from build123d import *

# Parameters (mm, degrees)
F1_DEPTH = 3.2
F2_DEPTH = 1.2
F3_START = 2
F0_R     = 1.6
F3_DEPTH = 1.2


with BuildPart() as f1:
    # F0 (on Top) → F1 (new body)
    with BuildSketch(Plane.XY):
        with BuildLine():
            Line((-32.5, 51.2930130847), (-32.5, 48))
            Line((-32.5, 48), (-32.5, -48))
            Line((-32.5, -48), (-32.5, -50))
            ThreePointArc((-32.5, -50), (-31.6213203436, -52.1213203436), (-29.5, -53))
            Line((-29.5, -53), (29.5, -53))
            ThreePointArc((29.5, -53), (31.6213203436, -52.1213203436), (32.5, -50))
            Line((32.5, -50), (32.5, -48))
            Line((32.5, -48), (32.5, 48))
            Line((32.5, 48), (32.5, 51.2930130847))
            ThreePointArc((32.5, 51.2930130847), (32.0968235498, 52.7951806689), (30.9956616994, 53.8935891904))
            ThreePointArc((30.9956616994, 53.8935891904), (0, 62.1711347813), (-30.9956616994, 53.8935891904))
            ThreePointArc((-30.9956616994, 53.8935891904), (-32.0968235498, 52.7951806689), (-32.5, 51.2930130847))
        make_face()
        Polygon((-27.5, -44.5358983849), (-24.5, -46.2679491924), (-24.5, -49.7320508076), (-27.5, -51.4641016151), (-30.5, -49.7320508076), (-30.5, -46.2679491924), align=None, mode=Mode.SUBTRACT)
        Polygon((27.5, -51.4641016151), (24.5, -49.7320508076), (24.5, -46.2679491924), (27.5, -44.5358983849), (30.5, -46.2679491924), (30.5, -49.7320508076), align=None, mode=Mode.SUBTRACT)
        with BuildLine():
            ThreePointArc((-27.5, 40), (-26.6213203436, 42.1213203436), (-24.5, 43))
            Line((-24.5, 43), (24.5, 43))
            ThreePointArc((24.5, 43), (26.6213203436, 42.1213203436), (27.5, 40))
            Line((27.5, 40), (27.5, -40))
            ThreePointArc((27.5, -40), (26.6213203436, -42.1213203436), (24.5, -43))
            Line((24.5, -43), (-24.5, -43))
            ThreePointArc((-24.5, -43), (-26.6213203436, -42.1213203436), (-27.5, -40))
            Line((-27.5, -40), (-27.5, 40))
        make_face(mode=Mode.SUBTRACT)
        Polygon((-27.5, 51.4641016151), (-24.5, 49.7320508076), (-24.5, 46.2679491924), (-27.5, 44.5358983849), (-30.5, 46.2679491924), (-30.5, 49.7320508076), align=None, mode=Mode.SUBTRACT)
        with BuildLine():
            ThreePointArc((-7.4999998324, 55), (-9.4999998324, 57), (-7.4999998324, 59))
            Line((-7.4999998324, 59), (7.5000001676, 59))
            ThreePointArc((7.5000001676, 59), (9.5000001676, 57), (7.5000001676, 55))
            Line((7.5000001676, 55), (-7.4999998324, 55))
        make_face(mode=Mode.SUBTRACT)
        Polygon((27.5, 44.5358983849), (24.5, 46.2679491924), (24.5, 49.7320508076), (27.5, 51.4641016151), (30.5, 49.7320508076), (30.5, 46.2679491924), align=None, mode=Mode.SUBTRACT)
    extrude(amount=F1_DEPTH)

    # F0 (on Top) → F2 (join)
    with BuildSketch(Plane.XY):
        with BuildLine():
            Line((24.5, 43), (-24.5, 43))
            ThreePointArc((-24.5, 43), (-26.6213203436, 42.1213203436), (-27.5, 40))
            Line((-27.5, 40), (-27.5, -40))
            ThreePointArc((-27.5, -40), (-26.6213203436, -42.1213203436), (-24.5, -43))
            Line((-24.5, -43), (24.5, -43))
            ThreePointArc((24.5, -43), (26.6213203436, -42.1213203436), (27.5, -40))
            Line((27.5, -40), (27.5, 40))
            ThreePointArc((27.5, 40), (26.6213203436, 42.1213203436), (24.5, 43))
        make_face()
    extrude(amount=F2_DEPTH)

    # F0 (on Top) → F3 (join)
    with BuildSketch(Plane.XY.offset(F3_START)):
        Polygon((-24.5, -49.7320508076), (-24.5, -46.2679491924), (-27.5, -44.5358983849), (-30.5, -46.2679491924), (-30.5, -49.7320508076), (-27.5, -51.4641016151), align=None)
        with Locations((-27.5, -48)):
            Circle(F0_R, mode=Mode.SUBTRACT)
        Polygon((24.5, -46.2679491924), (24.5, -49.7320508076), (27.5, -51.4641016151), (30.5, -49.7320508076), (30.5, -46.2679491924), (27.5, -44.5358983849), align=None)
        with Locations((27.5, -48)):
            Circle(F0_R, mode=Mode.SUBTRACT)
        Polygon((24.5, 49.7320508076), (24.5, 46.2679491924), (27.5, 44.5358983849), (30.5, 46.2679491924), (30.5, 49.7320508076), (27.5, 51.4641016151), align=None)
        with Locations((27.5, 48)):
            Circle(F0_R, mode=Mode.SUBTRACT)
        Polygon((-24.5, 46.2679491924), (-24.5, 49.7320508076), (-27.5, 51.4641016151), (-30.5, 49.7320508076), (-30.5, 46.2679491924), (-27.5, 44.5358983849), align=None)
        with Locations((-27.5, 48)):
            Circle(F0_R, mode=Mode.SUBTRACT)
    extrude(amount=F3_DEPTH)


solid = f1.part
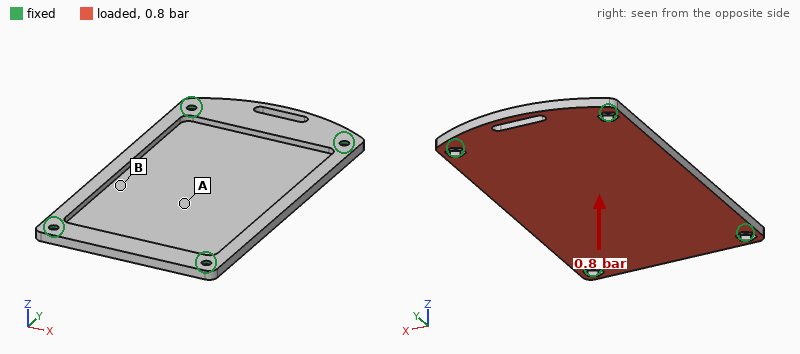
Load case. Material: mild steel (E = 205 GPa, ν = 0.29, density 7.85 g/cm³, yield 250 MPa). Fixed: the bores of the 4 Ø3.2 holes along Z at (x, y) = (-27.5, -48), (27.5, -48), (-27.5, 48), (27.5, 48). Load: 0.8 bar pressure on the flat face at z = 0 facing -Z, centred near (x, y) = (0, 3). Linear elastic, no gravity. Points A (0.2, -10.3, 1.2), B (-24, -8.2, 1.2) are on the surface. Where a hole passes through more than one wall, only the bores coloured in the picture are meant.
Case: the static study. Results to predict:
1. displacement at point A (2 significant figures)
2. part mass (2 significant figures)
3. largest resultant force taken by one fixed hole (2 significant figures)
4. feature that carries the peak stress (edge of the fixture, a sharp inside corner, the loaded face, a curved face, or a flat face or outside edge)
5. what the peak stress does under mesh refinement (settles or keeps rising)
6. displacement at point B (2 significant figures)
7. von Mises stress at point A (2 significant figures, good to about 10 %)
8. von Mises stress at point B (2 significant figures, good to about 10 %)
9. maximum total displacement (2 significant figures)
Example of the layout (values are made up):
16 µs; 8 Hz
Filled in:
0.18 mm; 100 g; 560 N; edge of the fixture; keeps rising; 0.13 mm; 38 MPa; 16 MPa; 0.20 mm
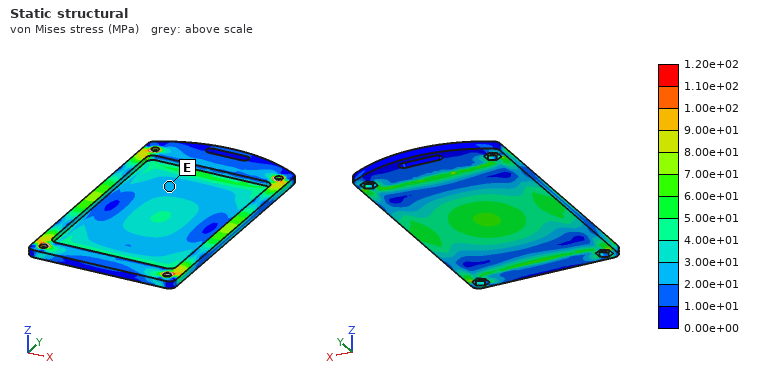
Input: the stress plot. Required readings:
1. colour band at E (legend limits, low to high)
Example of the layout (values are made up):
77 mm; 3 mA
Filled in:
2.00e+01 to 3.00e+01 MPa
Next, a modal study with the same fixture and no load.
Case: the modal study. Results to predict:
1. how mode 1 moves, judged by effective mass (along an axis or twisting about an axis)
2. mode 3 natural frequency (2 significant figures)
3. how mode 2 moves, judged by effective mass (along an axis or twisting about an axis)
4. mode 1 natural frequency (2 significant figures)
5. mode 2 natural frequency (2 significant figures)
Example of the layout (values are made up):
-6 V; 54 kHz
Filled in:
along Z; 2600 Hz; twisting about Y; 1200 Hz; 1700 Hz
